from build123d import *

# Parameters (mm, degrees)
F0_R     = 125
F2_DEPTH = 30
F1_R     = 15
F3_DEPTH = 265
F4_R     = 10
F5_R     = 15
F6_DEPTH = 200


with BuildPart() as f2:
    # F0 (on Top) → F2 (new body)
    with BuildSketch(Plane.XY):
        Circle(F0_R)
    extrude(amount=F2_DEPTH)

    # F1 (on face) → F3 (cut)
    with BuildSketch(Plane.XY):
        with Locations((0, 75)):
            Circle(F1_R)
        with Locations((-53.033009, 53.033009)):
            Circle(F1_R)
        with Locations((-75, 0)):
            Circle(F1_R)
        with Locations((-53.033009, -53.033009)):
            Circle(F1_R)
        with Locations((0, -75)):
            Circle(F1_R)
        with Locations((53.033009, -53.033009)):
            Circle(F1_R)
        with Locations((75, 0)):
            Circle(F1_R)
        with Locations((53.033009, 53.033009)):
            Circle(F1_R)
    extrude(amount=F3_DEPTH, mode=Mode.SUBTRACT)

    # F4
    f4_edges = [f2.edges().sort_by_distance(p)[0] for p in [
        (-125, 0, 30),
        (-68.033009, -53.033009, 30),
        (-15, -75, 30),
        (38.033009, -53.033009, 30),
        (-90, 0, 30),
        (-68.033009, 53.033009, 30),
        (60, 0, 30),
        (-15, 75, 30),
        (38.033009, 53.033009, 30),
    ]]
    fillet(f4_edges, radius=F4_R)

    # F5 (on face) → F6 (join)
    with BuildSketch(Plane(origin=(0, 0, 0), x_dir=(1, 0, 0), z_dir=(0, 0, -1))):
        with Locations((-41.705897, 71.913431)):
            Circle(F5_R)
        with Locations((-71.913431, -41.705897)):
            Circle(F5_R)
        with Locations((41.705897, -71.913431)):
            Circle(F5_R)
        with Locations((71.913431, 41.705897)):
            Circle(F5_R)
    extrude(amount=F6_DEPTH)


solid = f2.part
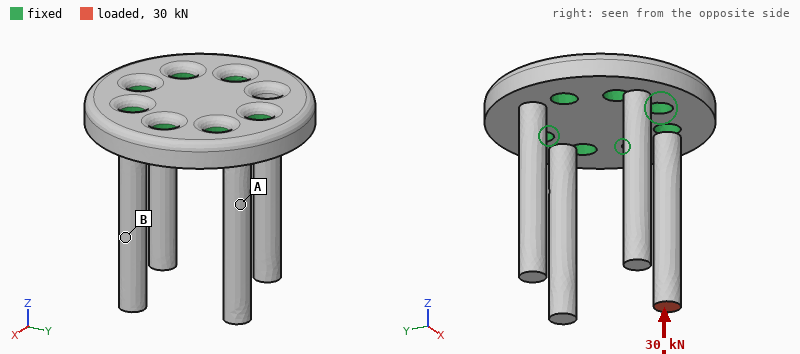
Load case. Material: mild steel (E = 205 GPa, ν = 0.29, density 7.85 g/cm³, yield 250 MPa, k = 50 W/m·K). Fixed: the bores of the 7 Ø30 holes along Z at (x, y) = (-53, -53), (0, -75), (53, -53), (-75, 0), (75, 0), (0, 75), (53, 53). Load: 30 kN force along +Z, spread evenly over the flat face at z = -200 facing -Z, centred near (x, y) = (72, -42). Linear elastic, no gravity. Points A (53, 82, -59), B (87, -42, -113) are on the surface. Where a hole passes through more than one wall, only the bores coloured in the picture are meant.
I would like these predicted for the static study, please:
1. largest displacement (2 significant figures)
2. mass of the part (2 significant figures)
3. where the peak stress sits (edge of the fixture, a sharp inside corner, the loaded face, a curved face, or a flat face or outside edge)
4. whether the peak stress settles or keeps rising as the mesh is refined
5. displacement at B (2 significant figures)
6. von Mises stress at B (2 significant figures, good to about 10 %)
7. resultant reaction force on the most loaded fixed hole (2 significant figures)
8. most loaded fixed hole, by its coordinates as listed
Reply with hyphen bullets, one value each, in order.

- 49 µm
- 14 kg
- edge of the fixture
- keeps rising
- 29 µm
- 42 MPa
- 24 kN
- (53, -53)
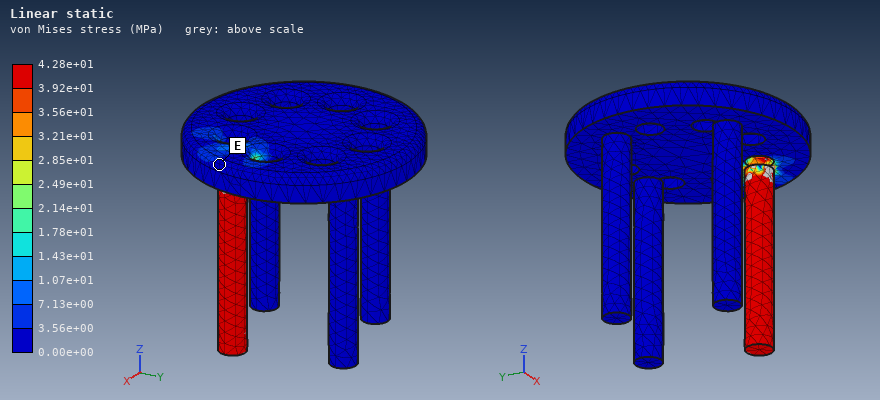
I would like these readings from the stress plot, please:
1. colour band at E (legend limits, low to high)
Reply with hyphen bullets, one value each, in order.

- 0.00e+00 to 3.56e+00 MPa
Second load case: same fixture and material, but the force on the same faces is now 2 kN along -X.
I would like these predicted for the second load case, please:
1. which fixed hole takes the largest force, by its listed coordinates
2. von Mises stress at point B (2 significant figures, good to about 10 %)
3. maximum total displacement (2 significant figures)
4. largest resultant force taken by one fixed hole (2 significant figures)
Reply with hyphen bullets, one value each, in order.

- (75, 0)
- 66 MPa
- 0.77 mm
- 7.1 kN
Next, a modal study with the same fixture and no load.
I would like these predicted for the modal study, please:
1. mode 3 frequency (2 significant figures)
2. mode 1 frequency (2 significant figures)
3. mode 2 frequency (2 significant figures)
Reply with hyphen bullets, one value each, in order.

- 480 Hz
- 450 Hz
- 470 Hz
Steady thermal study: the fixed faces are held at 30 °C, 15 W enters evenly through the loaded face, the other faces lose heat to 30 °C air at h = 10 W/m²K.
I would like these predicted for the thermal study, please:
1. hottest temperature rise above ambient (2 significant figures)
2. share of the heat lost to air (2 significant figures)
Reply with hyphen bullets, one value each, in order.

- 65 K
- 39 %
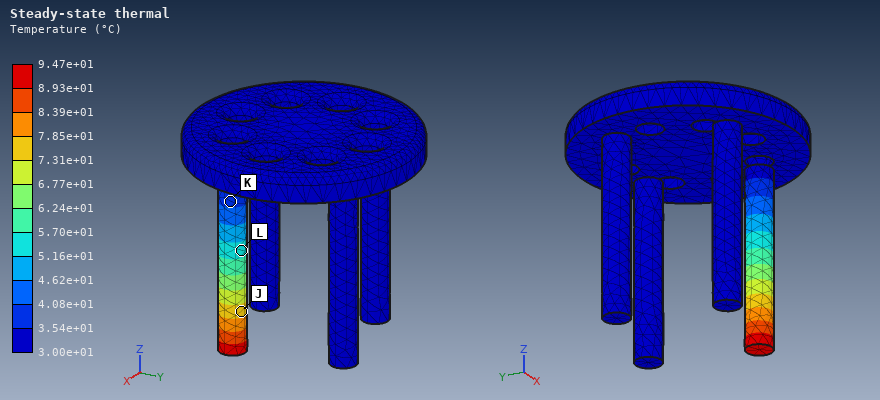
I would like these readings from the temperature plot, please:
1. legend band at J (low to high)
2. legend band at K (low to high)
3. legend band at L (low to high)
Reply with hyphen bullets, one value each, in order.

- 7.31e+01 to 7.85e+01 °C
- 3.54e+01 to 4.08e+01 °C
- 5.16e+01 to 5.70e+01 °C
